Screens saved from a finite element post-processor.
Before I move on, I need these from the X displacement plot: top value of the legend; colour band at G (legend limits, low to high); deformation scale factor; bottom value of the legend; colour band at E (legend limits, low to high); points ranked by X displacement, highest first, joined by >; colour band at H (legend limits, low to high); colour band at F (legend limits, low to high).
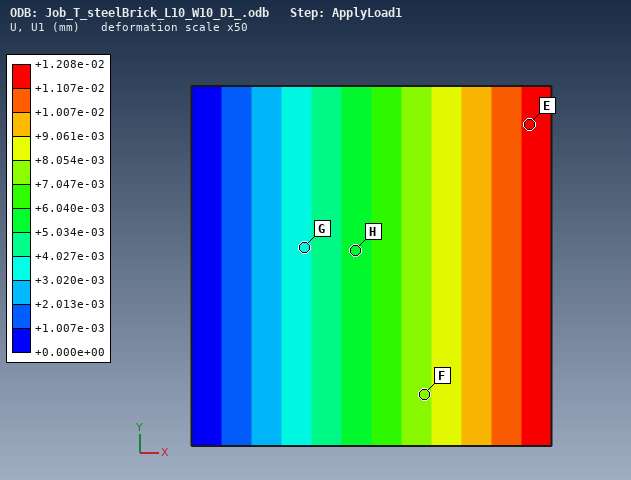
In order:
+1.208e-02 mm
+3.020e-03 to +4.027e-03 mm
50
+0.000e+00 mm
+1.107e-02 to +1.208e-02 mm
E > F > H > G
+5.034e-03 to +6.040e-03 mm
+7.047e-03 to +8.054e-03 mm
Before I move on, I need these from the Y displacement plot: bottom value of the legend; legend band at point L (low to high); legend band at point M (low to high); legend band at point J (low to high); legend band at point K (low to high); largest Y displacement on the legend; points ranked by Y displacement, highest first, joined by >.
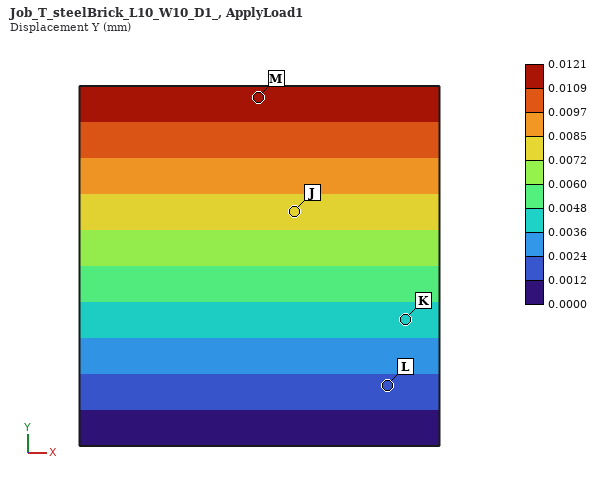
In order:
0.0000 mm
0.0012 to 0.0024 mm
0.0109 to 0.0121 mm
0.0072 to 0.0085 mm
0.0036 to 0.0048 mm
0.0121 mm
M > J > K > L
